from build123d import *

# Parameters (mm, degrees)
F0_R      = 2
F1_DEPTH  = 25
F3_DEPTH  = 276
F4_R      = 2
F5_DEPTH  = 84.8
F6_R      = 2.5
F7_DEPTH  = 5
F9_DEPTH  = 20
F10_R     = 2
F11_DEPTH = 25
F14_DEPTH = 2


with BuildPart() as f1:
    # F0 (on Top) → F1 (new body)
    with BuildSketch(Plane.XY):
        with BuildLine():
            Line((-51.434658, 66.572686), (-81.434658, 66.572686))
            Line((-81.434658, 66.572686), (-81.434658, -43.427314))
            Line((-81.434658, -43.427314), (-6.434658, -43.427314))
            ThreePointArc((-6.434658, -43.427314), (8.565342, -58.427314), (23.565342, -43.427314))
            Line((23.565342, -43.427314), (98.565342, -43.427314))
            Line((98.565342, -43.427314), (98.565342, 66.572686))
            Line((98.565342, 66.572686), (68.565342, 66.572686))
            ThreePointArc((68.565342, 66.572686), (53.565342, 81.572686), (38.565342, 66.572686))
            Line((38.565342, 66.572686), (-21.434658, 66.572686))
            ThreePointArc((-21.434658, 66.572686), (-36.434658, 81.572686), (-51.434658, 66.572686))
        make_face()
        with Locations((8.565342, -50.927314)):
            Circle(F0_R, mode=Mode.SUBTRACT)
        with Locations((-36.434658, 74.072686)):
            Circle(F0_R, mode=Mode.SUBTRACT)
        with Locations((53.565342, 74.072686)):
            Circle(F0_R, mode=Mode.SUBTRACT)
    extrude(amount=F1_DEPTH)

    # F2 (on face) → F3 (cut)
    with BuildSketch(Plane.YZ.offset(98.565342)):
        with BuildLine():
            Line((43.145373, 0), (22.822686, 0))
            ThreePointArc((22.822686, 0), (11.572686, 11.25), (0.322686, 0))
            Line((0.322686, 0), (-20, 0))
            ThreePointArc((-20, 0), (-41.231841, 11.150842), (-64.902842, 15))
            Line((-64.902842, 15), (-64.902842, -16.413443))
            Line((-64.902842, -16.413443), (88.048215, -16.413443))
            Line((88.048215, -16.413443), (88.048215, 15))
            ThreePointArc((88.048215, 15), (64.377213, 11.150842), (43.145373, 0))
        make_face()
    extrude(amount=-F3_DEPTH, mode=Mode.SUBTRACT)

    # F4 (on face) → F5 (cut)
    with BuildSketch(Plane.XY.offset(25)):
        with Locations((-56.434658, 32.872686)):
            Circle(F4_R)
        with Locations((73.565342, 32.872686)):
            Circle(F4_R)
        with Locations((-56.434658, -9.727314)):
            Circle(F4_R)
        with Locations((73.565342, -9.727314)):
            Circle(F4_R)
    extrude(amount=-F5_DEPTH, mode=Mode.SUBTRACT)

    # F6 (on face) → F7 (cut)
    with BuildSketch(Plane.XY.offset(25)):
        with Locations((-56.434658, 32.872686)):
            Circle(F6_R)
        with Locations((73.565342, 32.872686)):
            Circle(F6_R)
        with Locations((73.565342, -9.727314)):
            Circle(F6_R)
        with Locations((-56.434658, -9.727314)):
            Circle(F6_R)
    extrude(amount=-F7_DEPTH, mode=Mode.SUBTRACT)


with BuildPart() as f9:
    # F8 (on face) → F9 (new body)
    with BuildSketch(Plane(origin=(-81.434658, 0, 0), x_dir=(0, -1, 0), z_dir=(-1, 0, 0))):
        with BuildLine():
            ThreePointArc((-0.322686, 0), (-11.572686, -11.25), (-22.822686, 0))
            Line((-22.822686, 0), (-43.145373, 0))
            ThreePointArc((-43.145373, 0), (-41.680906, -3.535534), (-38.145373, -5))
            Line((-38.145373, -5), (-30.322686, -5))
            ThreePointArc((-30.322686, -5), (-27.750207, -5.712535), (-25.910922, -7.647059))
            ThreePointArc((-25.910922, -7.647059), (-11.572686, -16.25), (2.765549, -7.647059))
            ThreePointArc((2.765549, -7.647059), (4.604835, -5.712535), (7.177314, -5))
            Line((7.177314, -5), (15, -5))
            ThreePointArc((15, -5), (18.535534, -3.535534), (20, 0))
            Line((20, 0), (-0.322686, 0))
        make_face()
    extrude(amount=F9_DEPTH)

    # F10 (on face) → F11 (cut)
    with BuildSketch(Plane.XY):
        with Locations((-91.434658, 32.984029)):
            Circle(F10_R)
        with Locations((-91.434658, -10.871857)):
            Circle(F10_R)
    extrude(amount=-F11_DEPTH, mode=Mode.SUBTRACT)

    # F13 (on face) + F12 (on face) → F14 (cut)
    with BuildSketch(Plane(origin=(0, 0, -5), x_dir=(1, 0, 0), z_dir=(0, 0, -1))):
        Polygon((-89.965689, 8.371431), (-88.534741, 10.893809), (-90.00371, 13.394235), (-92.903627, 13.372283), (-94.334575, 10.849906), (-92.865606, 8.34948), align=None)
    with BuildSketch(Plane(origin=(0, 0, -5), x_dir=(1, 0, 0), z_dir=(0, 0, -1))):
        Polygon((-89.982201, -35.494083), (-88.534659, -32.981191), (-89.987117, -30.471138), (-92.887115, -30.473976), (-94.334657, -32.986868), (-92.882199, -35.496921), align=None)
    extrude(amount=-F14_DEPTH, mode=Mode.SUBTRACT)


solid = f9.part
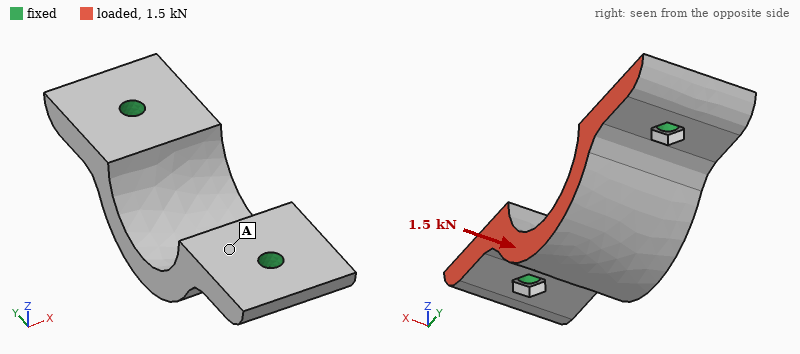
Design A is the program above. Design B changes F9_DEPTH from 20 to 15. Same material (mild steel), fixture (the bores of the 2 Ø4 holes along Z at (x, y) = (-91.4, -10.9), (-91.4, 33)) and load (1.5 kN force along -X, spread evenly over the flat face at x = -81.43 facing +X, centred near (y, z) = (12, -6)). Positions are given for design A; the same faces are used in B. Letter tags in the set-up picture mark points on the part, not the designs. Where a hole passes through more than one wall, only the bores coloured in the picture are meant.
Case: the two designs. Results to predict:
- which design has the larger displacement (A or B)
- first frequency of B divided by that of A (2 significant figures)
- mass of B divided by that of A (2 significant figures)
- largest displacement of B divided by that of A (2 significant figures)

B
1.1
0.74
1.2
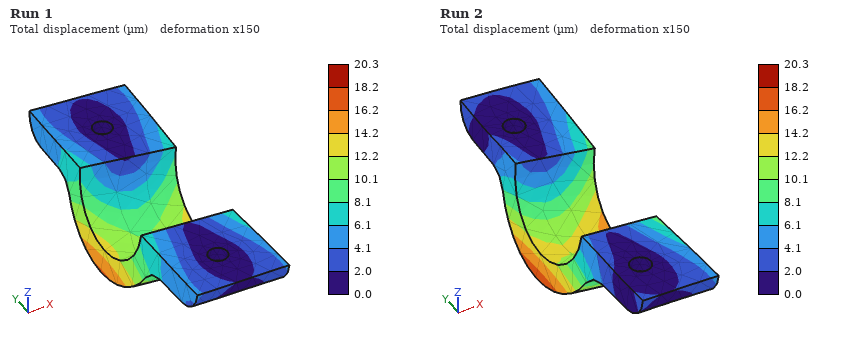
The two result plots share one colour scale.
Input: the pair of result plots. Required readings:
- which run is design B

Run 2
